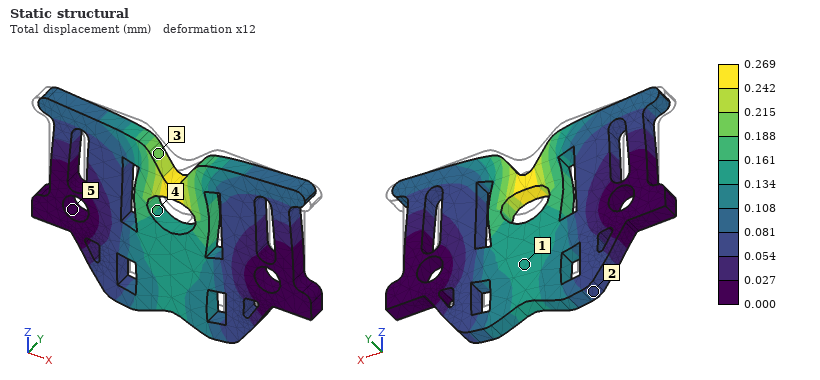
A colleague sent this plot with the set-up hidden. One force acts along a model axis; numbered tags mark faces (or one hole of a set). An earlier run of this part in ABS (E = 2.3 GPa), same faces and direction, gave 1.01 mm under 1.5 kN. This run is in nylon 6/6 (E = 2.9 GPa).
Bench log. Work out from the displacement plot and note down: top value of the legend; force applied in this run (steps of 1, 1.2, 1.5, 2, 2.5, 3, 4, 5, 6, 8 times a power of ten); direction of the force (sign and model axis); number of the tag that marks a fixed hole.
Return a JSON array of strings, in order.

["0.269 mm", "500 N", "-Z", "5"]
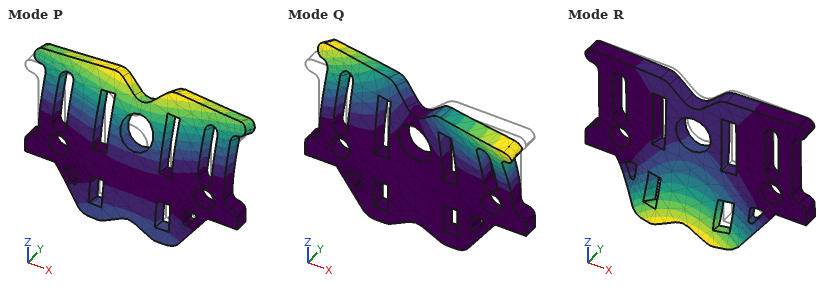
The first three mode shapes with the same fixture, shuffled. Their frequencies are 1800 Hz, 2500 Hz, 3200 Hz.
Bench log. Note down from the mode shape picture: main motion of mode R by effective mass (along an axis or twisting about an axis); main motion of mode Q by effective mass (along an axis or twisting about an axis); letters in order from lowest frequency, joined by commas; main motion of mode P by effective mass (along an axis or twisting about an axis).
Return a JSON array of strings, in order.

["along Y", "twisting about Z", "P, Q, R", "along Y"]
